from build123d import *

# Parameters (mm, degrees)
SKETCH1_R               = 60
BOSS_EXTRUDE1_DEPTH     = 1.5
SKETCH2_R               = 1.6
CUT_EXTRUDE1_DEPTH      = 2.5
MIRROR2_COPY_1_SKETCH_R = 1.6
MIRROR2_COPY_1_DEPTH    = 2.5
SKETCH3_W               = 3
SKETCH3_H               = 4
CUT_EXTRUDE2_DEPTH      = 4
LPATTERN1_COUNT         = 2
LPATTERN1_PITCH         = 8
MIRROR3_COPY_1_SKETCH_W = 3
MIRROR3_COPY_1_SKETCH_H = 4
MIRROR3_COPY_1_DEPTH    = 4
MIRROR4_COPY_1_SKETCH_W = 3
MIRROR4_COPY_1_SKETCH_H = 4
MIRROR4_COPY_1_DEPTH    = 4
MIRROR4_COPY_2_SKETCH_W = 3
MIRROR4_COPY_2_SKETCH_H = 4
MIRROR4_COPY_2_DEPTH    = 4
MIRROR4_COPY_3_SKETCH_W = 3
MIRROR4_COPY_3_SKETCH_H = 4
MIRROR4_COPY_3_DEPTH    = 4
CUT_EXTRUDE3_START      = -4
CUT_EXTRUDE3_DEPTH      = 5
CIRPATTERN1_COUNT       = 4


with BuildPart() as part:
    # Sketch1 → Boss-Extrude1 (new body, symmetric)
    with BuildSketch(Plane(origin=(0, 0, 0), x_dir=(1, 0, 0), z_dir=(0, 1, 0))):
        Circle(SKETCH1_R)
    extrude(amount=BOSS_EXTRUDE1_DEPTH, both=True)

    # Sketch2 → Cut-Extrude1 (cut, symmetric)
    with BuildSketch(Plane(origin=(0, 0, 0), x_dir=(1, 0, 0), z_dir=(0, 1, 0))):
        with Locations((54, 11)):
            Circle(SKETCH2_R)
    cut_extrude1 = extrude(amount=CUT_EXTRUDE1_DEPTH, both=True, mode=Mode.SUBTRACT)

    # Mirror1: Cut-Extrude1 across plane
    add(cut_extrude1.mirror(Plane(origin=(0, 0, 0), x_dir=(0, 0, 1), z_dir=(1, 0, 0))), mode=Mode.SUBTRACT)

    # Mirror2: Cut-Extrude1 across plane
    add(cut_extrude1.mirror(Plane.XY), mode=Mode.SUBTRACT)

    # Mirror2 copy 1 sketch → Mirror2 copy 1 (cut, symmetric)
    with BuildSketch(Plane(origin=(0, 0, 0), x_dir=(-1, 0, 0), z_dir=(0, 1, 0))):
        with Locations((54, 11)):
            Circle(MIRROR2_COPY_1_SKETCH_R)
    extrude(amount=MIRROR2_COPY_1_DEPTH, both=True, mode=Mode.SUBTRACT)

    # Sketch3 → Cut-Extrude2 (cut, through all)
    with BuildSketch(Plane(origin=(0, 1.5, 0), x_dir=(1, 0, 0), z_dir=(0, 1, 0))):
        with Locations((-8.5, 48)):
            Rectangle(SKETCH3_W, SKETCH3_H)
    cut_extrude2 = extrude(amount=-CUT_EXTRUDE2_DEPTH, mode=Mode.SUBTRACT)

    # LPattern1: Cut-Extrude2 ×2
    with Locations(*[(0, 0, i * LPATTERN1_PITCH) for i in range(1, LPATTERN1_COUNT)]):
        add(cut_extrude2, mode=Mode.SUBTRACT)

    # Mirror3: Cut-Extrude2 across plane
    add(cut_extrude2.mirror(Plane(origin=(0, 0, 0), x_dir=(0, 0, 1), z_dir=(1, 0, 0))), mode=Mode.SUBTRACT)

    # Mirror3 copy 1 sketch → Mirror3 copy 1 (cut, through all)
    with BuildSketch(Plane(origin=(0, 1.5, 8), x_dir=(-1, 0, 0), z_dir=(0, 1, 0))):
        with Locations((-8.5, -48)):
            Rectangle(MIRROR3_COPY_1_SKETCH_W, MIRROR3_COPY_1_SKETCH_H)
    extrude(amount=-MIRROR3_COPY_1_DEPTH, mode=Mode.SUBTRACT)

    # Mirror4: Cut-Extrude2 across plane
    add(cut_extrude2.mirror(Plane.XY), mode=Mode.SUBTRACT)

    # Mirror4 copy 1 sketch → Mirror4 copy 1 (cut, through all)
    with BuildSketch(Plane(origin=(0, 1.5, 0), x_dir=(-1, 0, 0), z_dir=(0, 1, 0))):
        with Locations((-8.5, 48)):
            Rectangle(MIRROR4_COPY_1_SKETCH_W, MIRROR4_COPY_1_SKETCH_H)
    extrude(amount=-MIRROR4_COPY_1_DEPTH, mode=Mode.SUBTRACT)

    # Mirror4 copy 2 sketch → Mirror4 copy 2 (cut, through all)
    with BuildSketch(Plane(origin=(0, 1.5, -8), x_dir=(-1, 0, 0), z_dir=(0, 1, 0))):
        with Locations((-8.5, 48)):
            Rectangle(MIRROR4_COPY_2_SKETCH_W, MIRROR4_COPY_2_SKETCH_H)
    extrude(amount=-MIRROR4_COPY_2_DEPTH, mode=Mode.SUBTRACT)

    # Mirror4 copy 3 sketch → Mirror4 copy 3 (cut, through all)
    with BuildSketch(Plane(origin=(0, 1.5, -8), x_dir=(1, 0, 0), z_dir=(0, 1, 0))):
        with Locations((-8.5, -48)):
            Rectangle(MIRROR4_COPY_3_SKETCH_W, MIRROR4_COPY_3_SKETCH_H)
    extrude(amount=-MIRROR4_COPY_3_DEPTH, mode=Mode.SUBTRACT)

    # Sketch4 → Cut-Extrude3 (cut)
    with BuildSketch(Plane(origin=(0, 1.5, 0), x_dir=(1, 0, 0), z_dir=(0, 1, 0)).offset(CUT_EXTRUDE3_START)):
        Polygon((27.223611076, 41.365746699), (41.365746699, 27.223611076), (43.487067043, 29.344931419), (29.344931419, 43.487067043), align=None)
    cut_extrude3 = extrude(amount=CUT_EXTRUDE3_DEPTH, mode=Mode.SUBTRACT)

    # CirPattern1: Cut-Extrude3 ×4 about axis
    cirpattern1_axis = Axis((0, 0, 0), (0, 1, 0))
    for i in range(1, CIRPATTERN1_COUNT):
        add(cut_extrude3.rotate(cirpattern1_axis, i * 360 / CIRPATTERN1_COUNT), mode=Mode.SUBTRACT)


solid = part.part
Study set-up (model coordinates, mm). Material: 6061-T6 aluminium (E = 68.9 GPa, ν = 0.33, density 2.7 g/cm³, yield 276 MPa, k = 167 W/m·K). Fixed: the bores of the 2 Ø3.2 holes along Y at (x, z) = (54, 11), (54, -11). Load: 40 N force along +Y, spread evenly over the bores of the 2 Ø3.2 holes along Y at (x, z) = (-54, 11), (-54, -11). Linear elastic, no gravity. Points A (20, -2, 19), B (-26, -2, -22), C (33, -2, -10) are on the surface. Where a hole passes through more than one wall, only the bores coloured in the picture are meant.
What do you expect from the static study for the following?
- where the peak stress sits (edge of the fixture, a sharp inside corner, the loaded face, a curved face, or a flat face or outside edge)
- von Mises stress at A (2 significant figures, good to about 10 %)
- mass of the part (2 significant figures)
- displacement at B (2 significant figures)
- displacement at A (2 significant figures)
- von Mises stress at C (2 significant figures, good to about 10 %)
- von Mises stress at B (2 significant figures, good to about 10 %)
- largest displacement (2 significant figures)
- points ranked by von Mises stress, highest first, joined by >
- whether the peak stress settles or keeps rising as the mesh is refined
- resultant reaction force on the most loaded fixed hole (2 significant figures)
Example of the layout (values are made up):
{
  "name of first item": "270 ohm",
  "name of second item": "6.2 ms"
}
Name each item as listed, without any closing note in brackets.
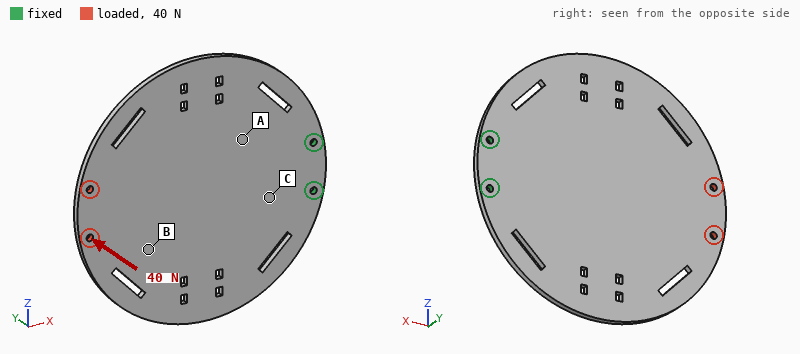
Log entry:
{
  "where the peak stress sits": "edge of the fixture",
  "von Mises stress at A": "18 MPa",
  "mass of the part": "89 g",
  "displacement at B": "0.96 mm",
  "displacement at A": "0.26 mm",
  "von Mises stress at C": "27 MPa",
  "von Mises stress at B": "8.5 MPa",
  "largest displacement": "1.6 mm",
  "points ranked by von Mises stress, highest first, joined by >": "C > A > B",
  "whether the peak stress settles or keeps rising as the mesh is refined": "keeps rising",
  "resultant reaction force on the most loaded fixed hole": "20 N"
}
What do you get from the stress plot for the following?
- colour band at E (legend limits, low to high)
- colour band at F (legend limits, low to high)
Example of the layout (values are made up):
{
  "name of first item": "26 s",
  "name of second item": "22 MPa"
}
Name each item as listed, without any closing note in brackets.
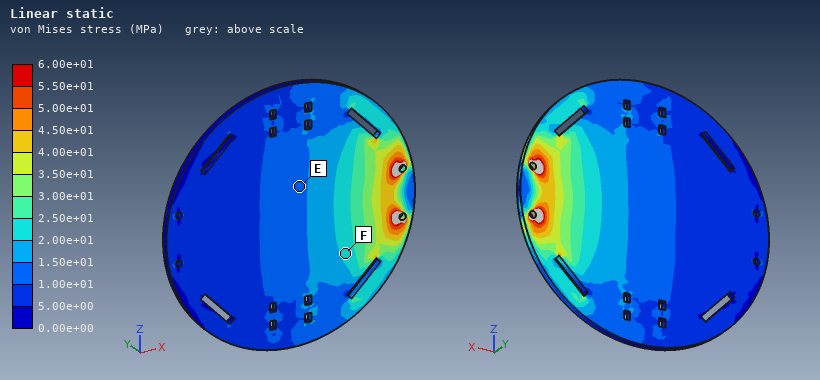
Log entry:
{
  "colour band at E": "1.00e+01 to 1.50e+01 MPa",
  "colour band at F": "2.00e+01 to 2.50e+01 MPa"
}
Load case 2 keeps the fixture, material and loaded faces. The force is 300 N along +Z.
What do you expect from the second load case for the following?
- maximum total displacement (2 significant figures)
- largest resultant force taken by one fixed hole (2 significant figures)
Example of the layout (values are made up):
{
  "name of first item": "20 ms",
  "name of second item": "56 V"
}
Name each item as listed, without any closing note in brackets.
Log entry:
{
  "maximum total displacement": "98 µm",
  "largest resultant force taken by one fixed hole": "1.3 kN"
}
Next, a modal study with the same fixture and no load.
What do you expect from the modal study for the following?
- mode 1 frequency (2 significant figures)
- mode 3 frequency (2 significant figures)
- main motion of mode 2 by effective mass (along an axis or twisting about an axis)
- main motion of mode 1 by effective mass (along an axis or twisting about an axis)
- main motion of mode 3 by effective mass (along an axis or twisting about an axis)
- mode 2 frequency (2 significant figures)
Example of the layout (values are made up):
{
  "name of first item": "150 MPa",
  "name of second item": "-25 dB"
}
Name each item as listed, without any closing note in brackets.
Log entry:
{
  "mode 1 frequency": "180 Hz",
  "mode 3 frequency": "910 Hz",
  "main motion of mode 2 by effective mass": "twisting about X",
  "main motion of mode 1 by effective mass": "along Y",
  "main motion of mode 3 by effective mass": "along Y",
  "mode 2 frequency": "390 Hz"
}
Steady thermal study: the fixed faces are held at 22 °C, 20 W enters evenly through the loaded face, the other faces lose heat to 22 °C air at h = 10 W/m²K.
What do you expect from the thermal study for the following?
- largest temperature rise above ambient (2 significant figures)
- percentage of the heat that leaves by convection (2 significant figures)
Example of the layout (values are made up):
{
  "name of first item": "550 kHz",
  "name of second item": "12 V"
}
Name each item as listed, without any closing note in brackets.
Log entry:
{
  "largest temperature rise above ambient": "55 K",
  "percentage of the heat that leaves by convection": "29 %"
}
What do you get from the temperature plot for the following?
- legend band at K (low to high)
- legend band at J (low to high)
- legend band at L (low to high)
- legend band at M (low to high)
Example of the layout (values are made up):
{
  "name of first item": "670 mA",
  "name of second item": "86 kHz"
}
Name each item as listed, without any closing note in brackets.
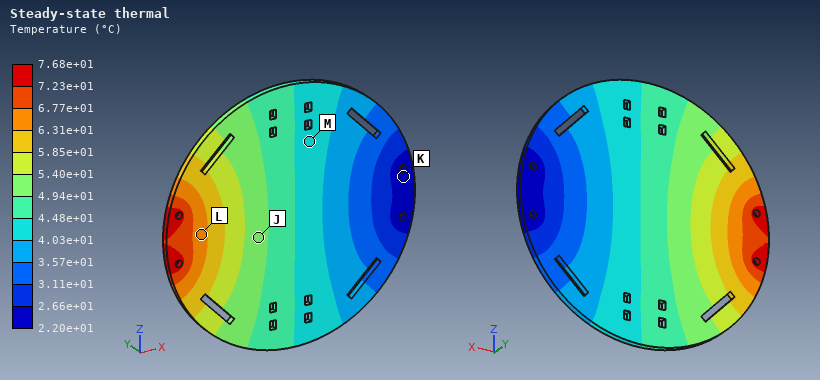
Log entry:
{
  "legend band at K": "2.20e+01 to 2.66e+01 °C",
  "legend band at J": "4.94e+01 to 5.40e+01 °C",
  "legend band at L": "6.31e+01 to 6.77e+01 °C",
  "legend band at M": "4.03e+01 to 4.48e+01 °C"
}
